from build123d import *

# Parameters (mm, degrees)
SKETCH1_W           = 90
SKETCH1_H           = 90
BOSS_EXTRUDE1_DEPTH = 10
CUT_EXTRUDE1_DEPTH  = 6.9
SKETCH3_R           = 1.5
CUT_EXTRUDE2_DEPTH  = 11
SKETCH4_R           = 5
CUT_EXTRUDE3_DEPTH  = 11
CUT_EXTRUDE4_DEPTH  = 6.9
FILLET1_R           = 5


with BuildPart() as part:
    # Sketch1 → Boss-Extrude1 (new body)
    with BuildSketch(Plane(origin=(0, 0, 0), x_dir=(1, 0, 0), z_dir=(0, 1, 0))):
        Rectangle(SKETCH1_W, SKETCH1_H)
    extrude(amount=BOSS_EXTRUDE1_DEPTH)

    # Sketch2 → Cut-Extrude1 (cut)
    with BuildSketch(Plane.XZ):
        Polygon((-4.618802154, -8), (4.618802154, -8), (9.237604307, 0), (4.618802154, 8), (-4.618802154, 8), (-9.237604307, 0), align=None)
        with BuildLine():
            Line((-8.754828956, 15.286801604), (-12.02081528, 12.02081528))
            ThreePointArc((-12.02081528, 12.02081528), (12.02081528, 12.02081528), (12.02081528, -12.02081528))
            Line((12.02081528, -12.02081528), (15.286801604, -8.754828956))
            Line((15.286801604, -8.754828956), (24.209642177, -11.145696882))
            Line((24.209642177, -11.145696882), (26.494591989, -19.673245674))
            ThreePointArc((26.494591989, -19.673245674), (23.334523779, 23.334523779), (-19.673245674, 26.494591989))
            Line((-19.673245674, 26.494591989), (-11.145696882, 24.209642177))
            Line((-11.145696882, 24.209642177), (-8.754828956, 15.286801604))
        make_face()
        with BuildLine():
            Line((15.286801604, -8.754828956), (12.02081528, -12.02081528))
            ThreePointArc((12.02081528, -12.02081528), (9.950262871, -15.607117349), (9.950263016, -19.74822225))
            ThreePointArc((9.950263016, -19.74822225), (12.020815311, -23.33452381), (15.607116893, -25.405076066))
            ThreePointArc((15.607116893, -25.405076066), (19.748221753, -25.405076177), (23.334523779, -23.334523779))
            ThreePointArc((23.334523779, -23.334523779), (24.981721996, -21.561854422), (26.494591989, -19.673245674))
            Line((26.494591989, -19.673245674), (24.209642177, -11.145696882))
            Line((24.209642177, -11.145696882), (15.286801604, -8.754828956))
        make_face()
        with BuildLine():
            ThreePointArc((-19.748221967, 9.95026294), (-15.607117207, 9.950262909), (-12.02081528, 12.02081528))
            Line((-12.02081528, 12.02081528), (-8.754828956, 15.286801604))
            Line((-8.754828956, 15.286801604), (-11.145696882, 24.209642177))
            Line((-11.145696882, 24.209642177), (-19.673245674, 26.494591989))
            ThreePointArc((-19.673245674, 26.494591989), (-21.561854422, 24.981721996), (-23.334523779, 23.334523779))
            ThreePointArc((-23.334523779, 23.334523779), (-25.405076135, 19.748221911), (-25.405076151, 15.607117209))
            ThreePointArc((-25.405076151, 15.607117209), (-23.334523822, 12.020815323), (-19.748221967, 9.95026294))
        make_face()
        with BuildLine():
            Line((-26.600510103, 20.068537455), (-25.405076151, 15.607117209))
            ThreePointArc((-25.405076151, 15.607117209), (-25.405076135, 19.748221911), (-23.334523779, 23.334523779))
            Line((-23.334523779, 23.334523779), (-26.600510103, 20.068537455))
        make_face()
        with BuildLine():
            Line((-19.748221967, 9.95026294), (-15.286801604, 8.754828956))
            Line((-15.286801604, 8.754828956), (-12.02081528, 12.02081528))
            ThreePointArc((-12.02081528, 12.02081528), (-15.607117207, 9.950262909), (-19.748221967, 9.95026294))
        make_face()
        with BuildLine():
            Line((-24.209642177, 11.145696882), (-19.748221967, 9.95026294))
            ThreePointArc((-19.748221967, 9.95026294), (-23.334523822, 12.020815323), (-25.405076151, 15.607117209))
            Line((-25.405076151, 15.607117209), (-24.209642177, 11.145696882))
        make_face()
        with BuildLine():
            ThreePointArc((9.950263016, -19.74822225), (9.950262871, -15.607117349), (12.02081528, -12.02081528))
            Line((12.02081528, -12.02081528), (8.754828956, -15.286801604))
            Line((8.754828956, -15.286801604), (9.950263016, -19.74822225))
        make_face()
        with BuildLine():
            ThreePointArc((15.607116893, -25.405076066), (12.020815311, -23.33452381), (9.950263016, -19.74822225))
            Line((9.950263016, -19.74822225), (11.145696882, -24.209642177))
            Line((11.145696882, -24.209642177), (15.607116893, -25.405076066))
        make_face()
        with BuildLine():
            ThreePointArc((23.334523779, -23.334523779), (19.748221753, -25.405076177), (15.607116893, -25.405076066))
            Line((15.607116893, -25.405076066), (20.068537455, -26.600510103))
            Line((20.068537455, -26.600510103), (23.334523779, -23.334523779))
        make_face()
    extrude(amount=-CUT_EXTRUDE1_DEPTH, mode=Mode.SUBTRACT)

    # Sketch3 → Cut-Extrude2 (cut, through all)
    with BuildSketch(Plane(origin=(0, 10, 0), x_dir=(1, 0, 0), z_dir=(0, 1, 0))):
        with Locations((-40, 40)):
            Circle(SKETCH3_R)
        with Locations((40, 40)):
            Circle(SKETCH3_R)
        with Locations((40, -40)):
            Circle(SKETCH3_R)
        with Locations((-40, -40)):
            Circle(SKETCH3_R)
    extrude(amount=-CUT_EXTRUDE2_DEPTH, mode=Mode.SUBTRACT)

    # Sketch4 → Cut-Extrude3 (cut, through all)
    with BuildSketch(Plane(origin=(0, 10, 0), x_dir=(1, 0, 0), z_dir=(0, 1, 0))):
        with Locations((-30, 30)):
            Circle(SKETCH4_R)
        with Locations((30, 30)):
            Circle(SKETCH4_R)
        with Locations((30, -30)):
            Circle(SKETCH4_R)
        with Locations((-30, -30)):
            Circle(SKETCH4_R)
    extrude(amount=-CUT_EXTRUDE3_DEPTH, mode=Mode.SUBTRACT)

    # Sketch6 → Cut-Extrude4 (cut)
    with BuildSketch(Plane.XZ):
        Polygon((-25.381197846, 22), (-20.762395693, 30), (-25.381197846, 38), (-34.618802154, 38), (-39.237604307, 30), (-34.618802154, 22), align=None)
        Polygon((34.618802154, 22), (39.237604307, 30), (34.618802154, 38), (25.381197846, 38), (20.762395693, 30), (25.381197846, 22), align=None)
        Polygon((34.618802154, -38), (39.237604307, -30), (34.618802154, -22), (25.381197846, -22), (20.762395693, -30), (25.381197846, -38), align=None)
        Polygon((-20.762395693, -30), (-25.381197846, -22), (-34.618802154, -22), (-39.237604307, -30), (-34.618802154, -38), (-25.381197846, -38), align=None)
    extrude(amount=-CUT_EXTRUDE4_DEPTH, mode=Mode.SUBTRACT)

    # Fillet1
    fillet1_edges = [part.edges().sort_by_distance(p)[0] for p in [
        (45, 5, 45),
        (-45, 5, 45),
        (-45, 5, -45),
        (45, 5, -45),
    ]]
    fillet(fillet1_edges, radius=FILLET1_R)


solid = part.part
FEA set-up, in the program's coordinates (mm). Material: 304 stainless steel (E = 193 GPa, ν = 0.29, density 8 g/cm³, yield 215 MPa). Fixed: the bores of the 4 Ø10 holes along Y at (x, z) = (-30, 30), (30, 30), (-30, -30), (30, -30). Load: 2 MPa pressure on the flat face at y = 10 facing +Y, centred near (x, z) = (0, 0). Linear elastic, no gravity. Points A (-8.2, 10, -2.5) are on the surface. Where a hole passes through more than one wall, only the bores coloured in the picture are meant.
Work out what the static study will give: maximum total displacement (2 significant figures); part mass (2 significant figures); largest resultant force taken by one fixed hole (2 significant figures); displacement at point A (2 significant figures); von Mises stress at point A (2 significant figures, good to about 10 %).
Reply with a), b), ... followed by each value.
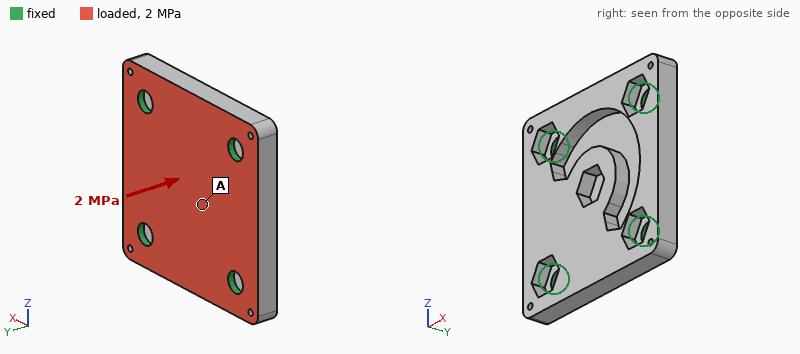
a) 40 µm
b) 490 g
c) 4.4 kN
d) 28 µm
e) 22 MPa
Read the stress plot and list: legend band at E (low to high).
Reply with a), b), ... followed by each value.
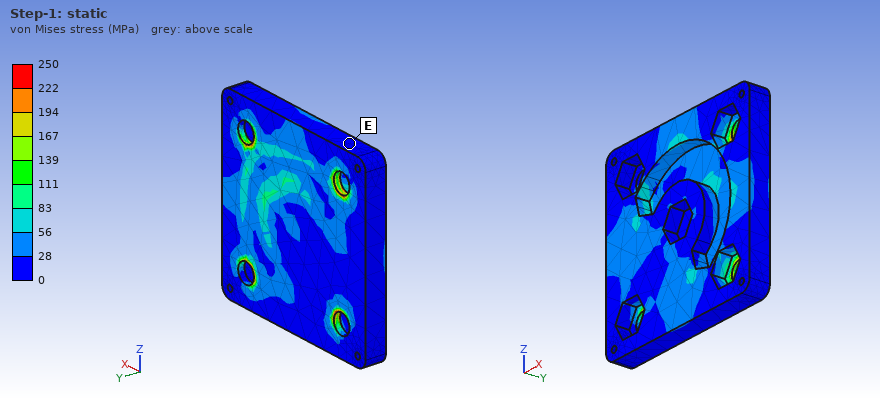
a) 0 to 28 MPa
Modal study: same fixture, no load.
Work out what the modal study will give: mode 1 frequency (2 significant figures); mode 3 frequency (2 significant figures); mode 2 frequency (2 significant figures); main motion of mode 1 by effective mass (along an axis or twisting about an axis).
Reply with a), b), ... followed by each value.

a) 6100 Hz
b) 8800 Hz
c) 7900 Hz
d) along Y
